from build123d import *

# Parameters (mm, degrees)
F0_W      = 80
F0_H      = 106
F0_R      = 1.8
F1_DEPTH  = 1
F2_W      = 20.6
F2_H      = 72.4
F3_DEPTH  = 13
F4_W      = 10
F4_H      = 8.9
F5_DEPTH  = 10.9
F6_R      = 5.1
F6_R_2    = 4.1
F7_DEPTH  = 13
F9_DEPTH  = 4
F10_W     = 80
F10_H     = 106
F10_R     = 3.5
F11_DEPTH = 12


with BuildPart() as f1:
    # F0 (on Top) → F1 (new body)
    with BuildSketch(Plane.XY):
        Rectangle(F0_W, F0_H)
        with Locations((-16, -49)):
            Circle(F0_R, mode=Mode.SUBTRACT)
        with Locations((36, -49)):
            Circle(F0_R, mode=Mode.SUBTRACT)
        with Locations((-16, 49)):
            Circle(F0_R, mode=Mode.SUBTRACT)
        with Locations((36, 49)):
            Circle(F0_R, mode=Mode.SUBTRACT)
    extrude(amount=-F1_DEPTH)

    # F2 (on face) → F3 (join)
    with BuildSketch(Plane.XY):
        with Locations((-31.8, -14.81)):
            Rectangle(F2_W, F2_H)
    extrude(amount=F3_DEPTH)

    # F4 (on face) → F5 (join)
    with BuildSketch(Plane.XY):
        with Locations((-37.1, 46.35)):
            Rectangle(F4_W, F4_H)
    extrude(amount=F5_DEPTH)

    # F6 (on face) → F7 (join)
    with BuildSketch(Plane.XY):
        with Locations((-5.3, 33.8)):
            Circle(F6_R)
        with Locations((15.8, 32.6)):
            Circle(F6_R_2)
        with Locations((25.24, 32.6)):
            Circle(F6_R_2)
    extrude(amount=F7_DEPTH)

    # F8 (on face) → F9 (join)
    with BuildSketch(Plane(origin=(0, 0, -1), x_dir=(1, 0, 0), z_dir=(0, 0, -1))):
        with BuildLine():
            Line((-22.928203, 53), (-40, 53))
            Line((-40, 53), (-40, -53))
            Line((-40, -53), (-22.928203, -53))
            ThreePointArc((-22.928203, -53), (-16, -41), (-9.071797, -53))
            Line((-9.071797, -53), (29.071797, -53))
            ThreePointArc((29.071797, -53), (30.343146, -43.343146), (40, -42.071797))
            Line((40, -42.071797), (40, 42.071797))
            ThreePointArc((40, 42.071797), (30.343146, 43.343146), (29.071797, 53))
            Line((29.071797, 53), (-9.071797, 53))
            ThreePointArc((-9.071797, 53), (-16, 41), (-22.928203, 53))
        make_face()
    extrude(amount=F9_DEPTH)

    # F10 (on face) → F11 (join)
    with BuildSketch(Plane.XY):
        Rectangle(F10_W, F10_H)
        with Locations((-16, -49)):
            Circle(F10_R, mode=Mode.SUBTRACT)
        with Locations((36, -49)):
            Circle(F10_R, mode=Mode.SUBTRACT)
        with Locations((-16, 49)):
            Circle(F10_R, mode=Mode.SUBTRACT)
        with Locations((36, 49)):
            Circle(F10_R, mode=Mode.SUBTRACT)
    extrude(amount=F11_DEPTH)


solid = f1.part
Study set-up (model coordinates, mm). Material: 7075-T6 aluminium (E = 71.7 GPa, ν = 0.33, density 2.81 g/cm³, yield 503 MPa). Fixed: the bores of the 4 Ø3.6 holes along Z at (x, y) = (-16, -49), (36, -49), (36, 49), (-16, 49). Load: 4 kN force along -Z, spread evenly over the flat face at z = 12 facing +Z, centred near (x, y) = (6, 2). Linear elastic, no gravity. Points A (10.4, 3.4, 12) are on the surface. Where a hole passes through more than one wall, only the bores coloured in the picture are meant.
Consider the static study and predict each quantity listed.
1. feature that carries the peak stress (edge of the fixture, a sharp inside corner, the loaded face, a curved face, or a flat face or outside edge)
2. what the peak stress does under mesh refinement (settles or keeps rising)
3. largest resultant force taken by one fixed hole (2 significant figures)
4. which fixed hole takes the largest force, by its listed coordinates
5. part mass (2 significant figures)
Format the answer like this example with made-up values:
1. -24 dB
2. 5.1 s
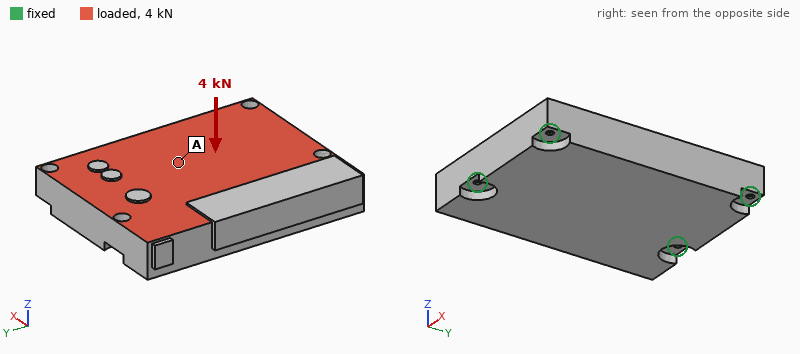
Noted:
1. edge of the fixture
2. keeps rising
3. 1.3 kN
4. (-16, 49)
5. 400 g
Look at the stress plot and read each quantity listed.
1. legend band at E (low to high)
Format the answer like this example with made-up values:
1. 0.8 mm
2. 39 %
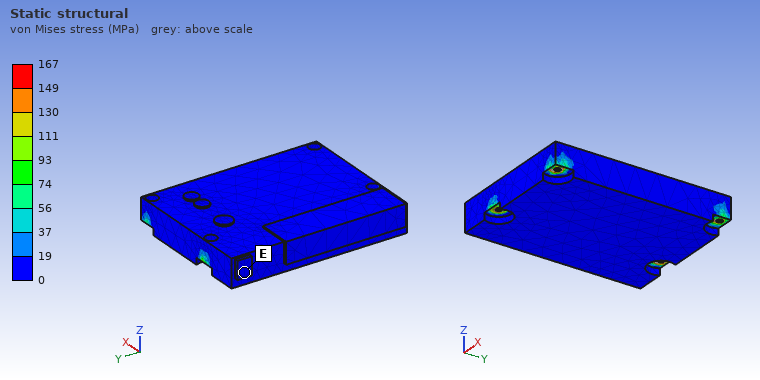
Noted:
1. 0 to 19 MPa
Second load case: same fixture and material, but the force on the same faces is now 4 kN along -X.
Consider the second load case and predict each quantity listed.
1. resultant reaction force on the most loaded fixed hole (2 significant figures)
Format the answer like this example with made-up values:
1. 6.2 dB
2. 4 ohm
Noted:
1. 1.3 kN
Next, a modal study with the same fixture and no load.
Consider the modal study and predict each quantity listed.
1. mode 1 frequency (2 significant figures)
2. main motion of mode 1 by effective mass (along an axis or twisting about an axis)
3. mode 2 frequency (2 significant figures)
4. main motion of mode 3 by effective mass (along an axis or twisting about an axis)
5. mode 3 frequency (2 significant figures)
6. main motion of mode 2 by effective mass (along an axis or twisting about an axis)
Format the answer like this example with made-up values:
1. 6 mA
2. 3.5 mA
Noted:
1. 2800 Hz
2. along Z
3. 3900 Hz
4. along Y
5. 5800 Hz
6. along Z
